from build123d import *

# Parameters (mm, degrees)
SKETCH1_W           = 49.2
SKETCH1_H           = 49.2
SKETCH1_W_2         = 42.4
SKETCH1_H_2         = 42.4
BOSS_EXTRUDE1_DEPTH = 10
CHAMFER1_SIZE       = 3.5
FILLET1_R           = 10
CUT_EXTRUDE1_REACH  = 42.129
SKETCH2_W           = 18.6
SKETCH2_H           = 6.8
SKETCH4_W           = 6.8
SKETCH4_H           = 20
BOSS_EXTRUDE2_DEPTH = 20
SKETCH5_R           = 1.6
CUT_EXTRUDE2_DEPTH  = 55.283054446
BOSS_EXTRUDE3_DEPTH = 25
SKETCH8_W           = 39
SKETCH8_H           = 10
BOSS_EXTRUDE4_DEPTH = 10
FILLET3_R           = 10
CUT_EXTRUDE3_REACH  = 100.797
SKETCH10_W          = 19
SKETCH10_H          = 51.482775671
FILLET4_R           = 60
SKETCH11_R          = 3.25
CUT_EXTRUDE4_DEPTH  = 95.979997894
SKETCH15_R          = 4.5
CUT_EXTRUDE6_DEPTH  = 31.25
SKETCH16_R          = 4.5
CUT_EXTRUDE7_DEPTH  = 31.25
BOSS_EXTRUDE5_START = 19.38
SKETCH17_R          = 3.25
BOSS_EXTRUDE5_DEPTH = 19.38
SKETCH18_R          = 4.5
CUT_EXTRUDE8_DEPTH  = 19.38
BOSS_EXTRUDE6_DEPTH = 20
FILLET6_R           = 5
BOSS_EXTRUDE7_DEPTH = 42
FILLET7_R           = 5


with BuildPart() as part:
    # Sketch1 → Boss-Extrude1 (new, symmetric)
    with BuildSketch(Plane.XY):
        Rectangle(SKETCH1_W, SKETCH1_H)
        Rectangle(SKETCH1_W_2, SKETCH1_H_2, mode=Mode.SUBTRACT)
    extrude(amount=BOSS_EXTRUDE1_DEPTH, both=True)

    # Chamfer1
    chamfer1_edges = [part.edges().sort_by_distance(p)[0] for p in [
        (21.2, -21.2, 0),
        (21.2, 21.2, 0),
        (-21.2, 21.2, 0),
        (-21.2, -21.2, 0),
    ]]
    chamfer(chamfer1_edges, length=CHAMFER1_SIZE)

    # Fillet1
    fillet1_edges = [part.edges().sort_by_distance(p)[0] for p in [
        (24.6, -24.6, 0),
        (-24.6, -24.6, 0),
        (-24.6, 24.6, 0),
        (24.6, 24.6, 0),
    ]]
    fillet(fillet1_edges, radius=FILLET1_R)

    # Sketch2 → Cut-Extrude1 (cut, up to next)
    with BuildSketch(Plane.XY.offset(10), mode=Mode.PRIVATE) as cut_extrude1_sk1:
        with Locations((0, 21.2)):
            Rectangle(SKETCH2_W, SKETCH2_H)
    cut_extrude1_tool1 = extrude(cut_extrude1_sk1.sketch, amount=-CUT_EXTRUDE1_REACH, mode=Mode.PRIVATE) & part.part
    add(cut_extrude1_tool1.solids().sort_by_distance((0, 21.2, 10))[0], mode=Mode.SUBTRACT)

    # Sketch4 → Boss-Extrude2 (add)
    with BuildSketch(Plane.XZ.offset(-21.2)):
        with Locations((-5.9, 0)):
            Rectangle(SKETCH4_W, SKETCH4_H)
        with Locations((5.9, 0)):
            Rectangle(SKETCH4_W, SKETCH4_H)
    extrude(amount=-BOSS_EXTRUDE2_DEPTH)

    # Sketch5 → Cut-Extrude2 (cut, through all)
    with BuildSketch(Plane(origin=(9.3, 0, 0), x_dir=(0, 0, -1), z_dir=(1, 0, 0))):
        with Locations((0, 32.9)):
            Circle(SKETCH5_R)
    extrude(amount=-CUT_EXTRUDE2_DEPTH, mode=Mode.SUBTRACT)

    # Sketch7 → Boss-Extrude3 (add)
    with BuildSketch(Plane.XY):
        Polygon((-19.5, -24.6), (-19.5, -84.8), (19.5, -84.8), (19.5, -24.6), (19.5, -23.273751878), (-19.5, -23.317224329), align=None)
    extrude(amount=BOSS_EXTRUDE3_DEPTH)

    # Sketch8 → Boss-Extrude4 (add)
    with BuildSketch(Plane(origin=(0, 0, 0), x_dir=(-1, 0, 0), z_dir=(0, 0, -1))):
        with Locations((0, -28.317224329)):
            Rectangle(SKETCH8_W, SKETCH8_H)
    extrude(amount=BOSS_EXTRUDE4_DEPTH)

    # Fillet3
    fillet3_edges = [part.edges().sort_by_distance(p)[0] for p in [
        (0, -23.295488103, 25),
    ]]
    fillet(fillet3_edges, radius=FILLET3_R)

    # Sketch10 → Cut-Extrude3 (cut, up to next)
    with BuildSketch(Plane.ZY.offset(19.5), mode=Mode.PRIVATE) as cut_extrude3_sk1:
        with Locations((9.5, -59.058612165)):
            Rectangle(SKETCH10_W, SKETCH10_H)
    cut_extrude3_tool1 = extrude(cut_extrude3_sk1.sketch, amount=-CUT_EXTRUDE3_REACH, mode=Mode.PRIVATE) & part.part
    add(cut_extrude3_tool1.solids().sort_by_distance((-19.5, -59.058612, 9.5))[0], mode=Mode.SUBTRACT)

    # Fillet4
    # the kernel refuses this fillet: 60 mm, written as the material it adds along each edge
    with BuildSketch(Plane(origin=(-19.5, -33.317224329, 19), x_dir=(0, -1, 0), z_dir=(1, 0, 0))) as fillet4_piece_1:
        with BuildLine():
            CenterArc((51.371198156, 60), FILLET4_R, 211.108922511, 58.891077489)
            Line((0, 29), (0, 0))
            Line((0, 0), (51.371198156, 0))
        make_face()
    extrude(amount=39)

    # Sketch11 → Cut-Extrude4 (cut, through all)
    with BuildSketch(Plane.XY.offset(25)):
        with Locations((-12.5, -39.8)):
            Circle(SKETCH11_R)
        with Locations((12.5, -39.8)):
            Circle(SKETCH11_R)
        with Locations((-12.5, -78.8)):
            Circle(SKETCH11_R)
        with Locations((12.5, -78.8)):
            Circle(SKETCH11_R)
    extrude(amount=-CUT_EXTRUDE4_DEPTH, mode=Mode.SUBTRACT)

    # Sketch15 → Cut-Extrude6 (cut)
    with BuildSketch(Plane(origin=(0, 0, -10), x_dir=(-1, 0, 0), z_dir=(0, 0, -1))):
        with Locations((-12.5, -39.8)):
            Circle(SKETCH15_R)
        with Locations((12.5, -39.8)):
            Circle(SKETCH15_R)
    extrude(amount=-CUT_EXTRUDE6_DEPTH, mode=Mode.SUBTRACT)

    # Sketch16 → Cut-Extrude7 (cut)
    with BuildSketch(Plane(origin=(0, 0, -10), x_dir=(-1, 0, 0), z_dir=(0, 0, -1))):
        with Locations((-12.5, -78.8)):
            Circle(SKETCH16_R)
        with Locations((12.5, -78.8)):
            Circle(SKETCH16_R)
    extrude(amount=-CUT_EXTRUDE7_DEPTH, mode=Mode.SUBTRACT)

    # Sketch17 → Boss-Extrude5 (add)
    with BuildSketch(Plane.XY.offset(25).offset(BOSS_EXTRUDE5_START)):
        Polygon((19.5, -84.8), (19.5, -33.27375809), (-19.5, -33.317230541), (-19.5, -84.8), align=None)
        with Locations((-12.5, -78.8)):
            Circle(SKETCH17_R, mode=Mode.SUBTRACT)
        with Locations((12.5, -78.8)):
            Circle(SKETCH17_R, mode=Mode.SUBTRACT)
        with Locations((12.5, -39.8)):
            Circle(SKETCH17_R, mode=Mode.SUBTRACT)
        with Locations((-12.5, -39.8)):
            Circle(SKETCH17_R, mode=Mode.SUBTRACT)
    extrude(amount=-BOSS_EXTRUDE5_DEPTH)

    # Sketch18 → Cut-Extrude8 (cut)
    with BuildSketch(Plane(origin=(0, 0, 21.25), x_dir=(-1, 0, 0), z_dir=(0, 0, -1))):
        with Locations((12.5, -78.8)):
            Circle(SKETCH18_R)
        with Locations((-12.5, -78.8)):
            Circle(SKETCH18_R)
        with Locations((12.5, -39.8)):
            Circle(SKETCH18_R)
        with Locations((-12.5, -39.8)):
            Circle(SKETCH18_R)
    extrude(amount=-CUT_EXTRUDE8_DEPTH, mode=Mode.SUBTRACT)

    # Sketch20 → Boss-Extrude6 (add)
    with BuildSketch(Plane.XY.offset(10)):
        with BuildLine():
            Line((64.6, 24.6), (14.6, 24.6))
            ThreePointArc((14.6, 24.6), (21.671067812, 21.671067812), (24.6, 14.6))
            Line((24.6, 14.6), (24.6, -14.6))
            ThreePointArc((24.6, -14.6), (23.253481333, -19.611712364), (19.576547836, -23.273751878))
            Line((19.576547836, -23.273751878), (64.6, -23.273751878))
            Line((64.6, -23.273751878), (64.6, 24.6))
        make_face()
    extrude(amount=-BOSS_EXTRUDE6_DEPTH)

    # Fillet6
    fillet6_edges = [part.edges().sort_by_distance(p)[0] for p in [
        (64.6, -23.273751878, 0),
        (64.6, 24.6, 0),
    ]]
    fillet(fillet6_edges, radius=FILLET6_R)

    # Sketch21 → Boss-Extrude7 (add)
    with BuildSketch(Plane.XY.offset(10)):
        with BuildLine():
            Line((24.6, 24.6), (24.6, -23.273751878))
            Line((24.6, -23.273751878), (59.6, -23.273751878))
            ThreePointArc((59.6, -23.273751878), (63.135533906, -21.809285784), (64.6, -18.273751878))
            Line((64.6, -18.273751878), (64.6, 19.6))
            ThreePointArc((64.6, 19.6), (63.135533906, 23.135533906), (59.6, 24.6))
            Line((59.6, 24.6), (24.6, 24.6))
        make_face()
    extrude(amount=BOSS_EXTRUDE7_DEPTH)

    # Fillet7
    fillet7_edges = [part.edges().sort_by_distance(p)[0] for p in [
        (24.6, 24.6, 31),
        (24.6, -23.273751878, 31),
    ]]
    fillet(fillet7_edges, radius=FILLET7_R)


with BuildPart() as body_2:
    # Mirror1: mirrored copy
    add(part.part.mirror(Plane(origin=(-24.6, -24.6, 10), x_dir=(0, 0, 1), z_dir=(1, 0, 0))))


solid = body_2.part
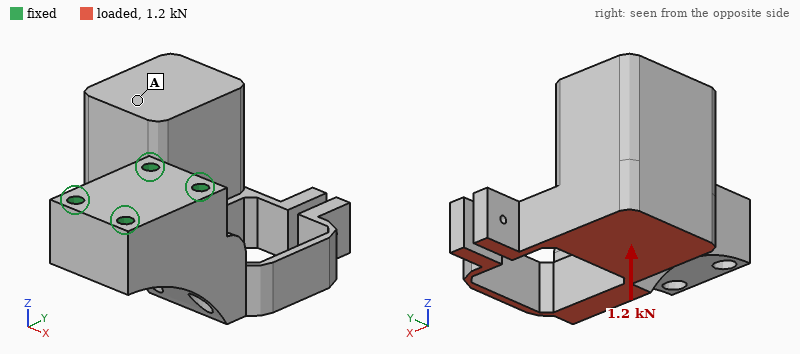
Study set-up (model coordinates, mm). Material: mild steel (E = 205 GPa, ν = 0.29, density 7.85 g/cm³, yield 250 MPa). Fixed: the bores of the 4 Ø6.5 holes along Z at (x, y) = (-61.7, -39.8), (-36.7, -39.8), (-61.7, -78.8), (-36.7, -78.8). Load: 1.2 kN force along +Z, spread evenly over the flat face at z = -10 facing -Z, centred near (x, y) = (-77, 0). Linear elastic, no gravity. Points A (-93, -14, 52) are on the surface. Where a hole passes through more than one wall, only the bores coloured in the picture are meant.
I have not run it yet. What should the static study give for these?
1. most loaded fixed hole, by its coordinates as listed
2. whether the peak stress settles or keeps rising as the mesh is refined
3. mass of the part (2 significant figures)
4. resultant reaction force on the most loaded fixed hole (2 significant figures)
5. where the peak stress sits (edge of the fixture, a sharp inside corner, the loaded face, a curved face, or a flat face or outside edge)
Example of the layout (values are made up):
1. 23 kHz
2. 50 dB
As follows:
1. (-61.7, -39.8)
2. keeps rising
3. 1.6 kg
4. 2.0 kN
5. a sharp inside corner
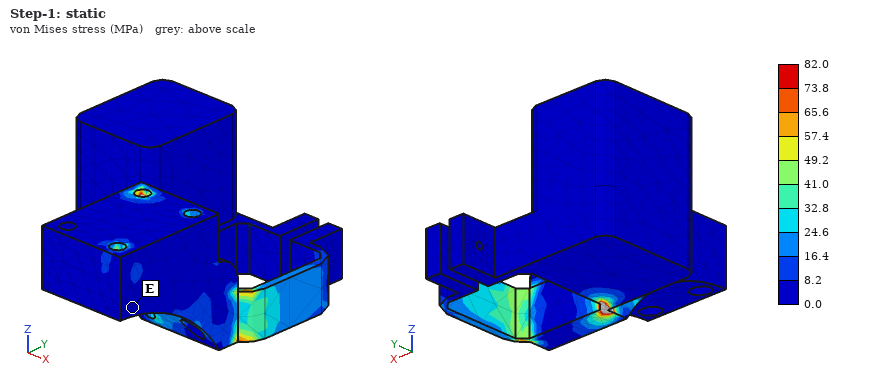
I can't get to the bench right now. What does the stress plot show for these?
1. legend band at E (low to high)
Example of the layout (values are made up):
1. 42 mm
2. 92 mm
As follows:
1. 0.0 to 8.2 MPa
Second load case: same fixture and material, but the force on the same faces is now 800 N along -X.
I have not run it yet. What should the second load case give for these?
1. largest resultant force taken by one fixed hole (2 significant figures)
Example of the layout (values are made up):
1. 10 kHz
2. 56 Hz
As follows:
1. 1.1 kN
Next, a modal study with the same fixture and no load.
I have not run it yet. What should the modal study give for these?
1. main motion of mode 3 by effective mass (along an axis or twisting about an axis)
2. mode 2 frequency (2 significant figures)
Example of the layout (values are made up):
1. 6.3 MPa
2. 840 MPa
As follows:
1. along Z
2. 400 Hz
